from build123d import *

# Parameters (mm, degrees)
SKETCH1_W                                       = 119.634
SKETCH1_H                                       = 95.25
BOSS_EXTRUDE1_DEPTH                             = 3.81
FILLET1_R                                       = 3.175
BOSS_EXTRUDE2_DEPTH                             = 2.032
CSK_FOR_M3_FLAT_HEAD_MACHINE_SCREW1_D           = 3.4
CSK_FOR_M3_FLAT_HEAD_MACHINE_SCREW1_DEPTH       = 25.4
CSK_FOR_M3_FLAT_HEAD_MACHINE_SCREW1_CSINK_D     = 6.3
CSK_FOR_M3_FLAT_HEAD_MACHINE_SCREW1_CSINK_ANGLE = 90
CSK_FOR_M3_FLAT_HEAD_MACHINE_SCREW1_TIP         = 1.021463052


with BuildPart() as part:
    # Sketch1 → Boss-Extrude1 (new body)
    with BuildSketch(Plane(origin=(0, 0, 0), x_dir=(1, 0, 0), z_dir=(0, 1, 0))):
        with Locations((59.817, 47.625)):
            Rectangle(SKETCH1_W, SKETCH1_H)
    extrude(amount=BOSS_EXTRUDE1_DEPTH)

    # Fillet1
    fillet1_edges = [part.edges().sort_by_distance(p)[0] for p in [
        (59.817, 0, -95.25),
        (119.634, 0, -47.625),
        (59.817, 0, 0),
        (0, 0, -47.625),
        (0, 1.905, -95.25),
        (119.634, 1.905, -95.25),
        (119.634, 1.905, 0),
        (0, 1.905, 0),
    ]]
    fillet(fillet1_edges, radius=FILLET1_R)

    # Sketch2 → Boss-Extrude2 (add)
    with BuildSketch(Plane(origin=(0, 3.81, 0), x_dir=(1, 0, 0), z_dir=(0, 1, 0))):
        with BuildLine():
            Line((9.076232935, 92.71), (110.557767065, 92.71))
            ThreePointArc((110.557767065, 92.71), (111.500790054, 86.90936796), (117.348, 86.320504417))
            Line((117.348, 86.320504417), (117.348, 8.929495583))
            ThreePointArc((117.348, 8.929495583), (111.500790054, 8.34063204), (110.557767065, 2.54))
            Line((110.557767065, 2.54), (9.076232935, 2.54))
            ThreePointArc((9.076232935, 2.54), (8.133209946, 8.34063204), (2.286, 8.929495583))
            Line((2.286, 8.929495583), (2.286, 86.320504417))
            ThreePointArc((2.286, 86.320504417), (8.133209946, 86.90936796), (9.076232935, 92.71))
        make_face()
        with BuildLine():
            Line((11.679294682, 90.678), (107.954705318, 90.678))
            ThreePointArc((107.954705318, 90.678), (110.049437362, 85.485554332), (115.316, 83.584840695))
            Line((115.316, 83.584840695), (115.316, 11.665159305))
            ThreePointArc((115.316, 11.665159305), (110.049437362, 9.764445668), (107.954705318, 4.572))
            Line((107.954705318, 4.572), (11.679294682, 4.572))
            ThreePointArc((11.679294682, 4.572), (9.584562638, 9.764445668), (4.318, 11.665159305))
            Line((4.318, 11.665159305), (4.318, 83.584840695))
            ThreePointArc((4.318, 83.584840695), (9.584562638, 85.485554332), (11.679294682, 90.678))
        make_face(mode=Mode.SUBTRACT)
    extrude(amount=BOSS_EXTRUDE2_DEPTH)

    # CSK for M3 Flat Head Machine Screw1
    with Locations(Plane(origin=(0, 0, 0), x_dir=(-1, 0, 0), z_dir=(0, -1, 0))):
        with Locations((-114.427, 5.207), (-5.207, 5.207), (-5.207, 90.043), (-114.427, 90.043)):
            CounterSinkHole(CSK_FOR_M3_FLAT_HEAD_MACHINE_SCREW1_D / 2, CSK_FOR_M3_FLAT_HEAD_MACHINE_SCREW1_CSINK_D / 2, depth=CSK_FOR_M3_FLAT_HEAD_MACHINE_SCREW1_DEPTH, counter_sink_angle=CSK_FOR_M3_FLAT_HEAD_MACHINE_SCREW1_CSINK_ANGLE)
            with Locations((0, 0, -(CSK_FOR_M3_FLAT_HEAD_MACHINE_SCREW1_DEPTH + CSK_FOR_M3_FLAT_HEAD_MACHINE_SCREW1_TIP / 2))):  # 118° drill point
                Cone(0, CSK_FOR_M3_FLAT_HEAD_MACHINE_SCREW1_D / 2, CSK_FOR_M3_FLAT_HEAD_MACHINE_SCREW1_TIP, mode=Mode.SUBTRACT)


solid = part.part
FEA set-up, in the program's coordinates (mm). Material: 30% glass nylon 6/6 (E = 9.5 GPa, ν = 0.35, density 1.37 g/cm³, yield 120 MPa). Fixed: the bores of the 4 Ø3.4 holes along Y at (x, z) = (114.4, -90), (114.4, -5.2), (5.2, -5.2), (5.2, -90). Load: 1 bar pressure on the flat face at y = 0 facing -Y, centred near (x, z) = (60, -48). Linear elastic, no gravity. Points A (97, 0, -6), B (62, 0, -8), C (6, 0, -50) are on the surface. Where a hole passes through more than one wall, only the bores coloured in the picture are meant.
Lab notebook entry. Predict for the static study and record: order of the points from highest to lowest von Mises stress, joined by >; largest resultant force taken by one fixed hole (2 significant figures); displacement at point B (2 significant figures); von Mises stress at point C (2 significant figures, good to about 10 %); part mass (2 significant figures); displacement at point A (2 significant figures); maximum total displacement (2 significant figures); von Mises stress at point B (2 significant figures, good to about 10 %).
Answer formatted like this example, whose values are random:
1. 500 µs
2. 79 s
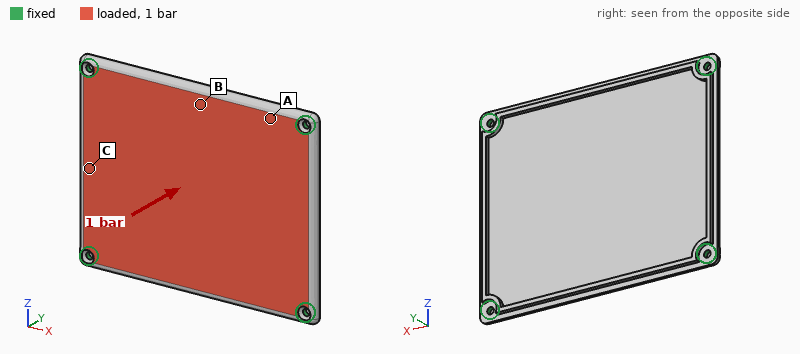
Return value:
1. B > C > A
2. 340 N
3. 1.4 mm
4. 19 MPa
5. 60 g
6. 0.53 mm
7. 1.8 mm
8. 29 MPa
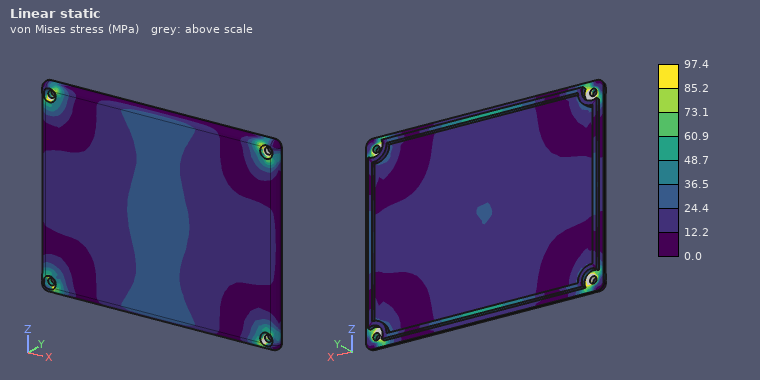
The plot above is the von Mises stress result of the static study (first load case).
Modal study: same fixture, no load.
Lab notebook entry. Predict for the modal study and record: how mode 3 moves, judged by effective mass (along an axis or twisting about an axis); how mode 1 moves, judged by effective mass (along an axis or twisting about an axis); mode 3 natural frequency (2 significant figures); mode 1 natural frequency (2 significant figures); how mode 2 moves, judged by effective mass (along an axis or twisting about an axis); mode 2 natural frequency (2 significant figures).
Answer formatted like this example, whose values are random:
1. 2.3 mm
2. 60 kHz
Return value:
1. twisting about Z
2. along Y
3. 1300 Hz
4. 600 Hz
5. twisting about X
6. 1000 Hz
